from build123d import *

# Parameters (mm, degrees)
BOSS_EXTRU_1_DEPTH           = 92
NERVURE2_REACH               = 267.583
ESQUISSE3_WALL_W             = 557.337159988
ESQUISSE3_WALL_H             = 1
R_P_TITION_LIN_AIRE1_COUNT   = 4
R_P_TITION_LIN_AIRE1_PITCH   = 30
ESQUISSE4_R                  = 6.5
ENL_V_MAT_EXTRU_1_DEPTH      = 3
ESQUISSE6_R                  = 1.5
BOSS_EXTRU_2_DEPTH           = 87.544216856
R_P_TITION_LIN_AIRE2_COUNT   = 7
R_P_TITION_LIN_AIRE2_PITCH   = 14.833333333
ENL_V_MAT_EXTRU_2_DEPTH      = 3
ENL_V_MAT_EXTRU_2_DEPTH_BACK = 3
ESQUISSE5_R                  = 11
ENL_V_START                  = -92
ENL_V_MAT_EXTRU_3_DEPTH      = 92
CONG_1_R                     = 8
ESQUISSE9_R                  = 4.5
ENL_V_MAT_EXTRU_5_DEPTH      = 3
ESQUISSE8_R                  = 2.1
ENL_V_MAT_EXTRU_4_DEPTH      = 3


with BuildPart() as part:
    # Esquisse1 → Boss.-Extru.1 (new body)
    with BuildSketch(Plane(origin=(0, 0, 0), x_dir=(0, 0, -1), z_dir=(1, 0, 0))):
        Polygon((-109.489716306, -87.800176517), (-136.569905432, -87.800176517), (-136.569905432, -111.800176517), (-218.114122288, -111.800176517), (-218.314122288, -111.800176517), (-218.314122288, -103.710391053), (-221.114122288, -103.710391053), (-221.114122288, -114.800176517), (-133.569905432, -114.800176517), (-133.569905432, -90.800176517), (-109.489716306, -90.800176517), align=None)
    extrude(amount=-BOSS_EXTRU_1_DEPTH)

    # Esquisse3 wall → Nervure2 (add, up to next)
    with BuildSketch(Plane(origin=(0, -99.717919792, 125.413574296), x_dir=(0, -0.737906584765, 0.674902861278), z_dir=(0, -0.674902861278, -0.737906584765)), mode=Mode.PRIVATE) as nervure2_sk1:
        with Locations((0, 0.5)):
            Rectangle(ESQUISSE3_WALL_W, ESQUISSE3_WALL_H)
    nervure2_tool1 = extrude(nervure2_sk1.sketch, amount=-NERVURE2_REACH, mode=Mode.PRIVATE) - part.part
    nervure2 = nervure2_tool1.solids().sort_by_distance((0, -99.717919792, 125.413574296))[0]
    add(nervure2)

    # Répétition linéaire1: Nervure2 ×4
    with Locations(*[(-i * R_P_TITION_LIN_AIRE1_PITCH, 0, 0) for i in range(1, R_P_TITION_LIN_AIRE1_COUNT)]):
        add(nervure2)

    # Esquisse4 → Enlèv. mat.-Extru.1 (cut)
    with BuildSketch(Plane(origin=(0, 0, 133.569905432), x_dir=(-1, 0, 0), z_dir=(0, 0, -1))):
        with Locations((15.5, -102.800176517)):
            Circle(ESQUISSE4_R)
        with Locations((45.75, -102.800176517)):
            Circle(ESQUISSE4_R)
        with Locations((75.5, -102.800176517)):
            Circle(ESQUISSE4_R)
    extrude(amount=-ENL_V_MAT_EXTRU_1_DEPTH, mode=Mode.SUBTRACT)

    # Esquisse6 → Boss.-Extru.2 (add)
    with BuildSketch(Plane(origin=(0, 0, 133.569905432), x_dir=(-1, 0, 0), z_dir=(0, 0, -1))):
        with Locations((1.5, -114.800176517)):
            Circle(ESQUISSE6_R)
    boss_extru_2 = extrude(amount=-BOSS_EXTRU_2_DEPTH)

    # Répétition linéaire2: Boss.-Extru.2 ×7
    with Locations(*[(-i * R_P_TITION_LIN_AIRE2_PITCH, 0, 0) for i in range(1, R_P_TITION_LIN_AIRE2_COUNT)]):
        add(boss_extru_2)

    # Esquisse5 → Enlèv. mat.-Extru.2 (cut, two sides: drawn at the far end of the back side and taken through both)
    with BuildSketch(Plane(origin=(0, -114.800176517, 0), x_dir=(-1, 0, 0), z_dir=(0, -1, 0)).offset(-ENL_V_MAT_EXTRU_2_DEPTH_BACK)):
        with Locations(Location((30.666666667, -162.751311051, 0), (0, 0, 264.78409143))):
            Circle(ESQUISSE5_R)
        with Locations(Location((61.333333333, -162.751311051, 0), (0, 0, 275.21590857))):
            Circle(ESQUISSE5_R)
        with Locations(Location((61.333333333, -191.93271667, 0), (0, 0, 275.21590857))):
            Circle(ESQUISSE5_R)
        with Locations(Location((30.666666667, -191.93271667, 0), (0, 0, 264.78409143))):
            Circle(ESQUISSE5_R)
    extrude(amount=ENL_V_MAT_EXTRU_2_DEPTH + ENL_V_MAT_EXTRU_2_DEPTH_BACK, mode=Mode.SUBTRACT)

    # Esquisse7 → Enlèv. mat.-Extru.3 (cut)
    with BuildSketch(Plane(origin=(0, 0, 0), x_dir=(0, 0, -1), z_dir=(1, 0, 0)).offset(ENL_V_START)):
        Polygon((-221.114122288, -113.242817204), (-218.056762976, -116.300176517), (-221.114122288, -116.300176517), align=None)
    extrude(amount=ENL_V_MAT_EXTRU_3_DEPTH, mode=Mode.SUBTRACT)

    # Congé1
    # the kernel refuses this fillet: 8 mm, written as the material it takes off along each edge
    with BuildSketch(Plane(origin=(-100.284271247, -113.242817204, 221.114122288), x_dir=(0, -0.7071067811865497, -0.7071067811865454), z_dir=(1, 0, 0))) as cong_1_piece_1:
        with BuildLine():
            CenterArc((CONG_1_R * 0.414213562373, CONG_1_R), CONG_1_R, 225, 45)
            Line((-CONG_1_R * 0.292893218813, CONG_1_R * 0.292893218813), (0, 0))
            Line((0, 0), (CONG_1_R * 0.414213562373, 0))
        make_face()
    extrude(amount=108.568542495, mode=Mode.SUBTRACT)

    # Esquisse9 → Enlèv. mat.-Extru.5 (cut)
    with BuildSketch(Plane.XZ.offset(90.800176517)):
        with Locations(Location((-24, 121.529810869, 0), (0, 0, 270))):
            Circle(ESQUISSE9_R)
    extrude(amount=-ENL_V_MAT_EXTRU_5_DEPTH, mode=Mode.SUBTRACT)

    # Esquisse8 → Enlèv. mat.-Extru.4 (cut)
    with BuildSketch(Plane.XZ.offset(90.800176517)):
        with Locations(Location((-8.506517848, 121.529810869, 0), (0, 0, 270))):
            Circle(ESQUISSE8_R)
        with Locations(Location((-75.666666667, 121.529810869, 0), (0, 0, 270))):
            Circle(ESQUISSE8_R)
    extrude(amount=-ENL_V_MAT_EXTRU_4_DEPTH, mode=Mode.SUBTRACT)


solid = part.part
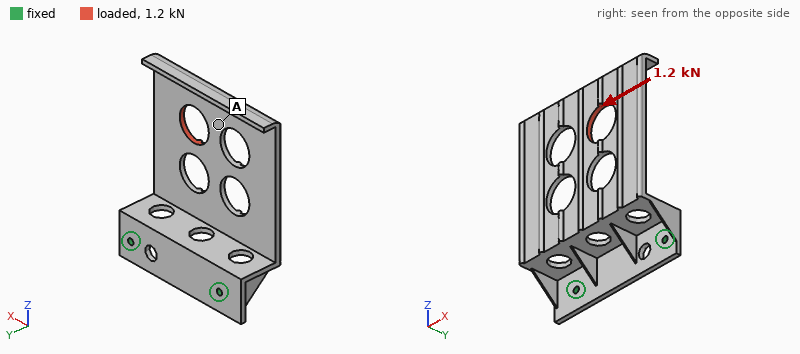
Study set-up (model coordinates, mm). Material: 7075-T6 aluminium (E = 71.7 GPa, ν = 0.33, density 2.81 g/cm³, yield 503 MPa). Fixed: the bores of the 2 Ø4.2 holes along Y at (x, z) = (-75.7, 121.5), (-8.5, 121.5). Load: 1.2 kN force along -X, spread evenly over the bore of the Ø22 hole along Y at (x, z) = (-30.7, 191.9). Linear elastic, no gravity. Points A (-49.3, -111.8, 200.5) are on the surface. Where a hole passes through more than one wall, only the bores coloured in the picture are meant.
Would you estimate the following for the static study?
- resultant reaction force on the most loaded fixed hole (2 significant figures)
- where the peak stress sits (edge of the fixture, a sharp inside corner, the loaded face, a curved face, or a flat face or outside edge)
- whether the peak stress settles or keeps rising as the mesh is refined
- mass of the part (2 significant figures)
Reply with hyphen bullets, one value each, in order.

- 1.4 kN
- edge of the fixture
- keeps rising
- 100 g
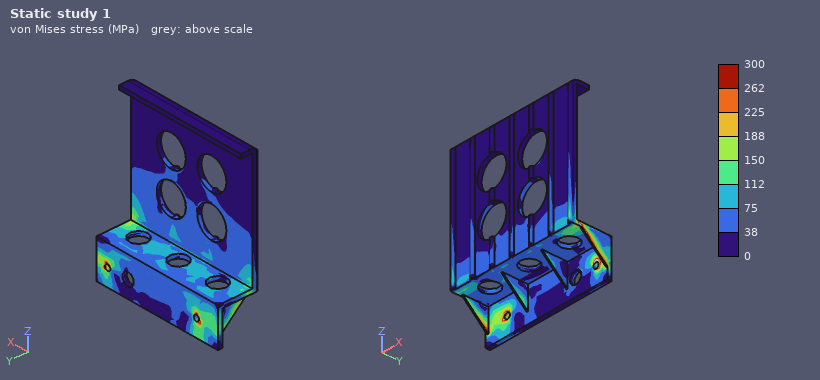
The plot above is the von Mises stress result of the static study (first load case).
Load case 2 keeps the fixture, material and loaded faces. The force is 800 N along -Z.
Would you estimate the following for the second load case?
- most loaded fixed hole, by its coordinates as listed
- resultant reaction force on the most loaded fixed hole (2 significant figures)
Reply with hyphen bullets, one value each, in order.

- (-8.5, 121.5)
- 520 N
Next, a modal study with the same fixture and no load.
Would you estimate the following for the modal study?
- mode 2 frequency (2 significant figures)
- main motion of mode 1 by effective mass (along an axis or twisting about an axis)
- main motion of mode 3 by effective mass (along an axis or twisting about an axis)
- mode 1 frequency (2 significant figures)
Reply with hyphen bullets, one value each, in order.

- 530 Hz
- along Y
- along X
- 210 Hz
